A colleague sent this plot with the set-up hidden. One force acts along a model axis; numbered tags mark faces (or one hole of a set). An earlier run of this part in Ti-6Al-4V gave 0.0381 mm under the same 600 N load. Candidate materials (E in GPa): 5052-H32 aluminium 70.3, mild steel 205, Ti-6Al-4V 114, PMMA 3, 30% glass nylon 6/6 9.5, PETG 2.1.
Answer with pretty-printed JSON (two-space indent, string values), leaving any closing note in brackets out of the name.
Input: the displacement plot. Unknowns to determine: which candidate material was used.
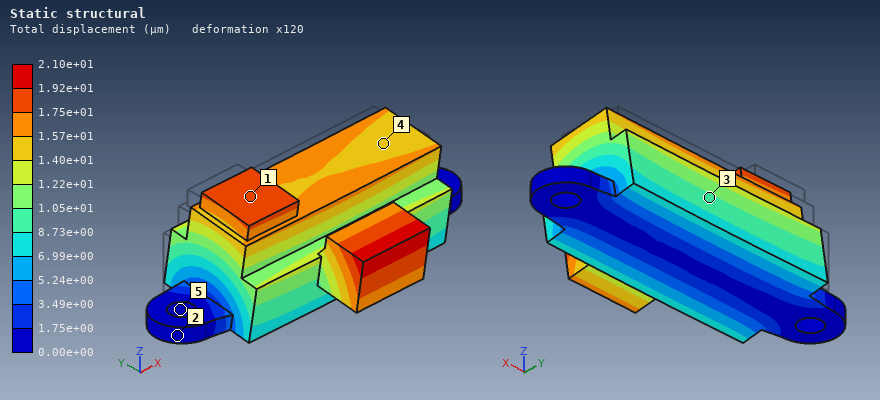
{
  "which candidate material was used": "mild steel"
}
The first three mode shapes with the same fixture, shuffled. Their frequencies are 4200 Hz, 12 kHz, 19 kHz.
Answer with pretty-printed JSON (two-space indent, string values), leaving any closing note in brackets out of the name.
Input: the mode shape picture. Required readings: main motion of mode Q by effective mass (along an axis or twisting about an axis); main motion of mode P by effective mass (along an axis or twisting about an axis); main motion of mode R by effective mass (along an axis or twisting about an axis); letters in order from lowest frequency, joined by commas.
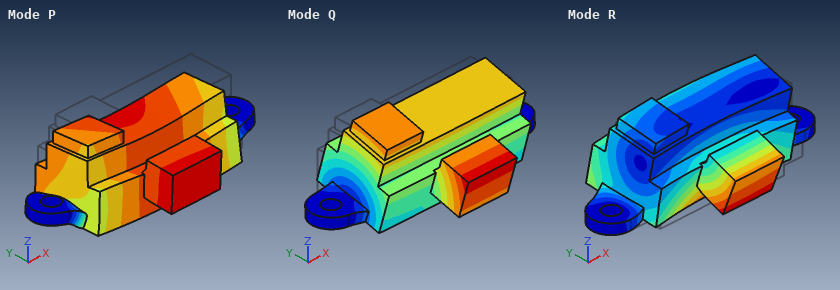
{
  "main motion of mode Q by effective mass": "along Y",
  "main motion of mode P by effective mass": "along Z",
  "main motion of mode R by effective mass": "along Y",
  "letters in order from lowest frequency, joined by commas": "Q, P, R"
}
